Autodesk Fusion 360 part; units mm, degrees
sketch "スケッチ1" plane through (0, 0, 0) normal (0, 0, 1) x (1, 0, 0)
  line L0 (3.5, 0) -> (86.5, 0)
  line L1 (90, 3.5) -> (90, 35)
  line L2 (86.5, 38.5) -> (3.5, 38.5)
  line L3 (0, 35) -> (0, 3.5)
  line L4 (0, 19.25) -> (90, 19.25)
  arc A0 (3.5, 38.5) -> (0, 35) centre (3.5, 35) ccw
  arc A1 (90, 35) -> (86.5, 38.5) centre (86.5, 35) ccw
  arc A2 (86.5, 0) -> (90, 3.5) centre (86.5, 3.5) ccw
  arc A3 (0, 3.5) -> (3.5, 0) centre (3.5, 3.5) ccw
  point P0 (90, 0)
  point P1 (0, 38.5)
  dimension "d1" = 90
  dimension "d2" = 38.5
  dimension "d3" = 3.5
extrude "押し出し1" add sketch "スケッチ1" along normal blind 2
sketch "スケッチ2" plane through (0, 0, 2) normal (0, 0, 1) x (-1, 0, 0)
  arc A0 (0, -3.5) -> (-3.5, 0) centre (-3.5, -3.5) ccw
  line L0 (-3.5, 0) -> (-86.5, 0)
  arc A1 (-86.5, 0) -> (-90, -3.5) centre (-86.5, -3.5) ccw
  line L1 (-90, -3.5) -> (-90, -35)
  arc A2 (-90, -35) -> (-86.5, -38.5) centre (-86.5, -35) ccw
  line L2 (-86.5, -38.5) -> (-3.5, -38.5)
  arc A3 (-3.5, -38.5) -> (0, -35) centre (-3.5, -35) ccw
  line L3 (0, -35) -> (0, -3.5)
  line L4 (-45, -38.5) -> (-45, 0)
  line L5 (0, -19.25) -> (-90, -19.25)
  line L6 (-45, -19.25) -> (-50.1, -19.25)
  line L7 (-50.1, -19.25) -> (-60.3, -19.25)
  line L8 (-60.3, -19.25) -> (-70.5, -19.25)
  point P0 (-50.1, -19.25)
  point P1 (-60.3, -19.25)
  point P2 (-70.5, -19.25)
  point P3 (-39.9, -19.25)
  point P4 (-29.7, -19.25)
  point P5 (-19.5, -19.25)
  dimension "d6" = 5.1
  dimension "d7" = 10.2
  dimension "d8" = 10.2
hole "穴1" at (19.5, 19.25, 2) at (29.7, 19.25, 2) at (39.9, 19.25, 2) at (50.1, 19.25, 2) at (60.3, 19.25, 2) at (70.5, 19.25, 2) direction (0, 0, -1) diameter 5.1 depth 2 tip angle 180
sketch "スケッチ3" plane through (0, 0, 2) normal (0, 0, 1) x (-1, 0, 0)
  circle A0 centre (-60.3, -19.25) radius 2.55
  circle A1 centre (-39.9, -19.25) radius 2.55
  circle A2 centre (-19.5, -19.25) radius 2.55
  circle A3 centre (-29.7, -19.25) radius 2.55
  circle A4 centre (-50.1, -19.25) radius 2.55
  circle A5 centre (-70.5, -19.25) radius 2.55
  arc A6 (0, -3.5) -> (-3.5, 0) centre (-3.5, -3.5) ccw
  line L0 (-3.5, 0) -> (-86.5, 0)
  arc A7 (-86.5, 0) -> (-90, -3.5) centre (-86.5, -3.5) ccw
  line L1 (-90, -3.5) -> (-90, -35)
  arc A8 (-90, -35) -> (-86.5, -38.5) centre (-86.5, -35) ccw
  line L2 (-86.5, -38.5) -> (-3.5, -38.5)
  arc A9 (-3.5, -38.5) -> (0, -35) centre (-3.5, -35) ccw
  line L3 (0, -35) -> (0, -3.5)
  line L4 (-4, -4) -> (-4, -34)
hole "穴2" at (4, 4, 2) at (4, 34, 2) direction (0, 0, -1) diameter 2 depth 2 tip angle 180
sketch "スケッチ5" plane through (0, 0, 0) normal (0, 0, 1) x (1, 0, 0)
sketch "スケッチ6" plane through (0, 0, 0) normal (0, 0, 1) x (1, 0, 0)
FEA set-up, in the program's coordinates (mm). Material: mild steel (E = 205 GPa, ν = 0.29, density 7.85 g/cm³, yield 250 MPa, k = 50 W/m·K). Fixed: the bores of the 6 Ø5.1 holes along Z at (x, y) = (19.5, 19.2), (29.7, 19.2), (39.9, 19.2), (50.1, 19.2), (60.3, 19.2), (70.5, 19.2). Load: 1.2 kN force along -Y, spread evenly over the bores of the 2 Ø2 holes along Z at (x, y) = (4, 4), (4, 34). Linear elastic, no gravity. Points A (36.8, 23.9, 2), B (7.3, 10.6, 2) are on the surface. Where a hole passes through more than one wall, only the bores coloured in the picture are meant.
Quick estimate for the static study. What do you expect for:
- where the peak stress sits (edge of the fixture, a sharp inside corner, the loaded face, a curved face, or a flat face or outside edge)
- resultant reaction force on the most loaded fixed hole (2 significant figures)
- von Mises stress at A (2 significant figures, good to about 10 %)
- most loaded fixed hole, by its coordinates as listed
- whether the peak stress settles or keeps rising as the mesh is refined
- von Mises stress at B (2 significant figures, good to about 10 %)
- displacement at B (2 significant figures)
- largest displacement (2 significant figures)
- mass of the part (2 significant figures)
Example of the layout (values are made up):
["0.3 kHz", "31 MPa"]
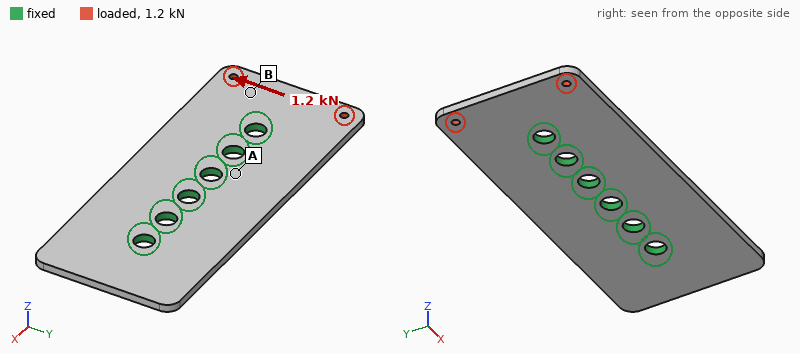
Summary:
["edge of the fixture", "1.6 kN", "14 MPa", "(19.5, 19.2)", "keeps rising", "32 MPa", "6.2 µm", "11 µm", "52 g"]
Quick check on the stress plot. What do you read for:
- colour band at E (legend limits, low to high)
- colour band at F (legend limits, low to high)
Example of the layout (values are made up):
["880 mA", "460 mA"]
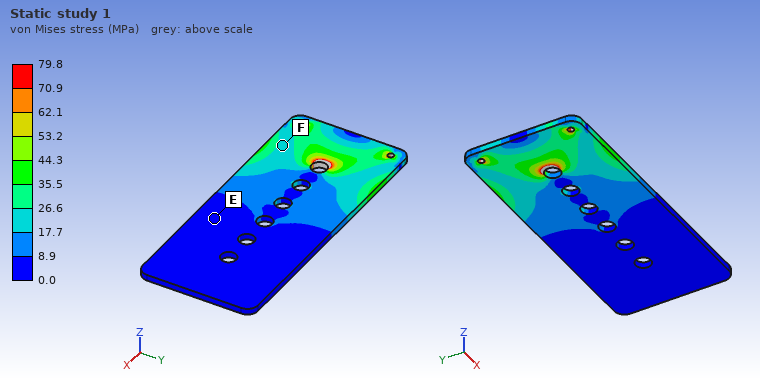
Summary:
["0.0 to 8.9 MPa", "17.7 to 26.6 MPa"]
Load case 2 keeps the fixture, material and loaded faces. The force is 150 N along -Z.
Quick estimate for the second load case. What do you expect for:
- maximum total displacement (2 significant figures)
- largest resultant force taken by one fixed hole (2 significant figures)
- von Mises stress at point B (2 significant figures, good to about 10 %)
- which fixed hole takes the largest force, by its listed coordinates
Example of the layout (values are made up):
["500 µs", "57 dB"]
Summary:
["74 µm", "210 N", "28 MPa", "(19.5, 19.2)"]
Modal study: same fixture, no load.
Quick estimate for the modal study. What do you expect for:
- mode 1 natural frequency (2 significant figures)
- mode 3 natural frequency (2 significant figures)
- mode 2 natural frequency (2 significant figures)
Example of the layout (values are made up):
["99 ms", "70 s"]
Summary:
["3900 Hz", "4000 Hz", "3900 Hz"]
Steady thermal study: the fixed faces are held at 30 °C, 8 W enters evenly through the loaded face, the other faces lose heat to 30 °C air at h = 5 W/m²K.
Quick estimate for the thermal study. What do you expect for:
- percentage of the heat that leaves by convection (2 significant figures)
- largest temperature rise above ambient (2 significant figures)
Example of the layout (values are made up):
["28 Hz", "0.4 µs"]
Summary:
["3.5 %", "57 K"]
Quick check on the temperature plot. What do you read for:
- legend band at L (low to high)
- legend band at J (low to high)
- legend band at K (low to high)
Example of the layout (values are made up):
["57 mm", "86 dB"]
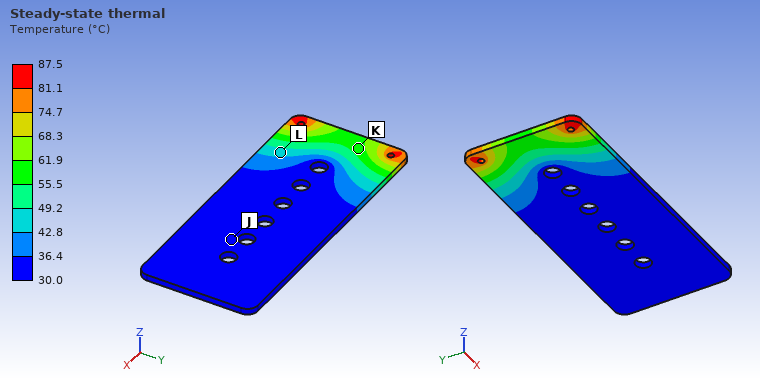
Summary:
["42.8 to 49.2 °C", "30.0 to 36.4 °C", "55.5 to 61.9 °C"]
